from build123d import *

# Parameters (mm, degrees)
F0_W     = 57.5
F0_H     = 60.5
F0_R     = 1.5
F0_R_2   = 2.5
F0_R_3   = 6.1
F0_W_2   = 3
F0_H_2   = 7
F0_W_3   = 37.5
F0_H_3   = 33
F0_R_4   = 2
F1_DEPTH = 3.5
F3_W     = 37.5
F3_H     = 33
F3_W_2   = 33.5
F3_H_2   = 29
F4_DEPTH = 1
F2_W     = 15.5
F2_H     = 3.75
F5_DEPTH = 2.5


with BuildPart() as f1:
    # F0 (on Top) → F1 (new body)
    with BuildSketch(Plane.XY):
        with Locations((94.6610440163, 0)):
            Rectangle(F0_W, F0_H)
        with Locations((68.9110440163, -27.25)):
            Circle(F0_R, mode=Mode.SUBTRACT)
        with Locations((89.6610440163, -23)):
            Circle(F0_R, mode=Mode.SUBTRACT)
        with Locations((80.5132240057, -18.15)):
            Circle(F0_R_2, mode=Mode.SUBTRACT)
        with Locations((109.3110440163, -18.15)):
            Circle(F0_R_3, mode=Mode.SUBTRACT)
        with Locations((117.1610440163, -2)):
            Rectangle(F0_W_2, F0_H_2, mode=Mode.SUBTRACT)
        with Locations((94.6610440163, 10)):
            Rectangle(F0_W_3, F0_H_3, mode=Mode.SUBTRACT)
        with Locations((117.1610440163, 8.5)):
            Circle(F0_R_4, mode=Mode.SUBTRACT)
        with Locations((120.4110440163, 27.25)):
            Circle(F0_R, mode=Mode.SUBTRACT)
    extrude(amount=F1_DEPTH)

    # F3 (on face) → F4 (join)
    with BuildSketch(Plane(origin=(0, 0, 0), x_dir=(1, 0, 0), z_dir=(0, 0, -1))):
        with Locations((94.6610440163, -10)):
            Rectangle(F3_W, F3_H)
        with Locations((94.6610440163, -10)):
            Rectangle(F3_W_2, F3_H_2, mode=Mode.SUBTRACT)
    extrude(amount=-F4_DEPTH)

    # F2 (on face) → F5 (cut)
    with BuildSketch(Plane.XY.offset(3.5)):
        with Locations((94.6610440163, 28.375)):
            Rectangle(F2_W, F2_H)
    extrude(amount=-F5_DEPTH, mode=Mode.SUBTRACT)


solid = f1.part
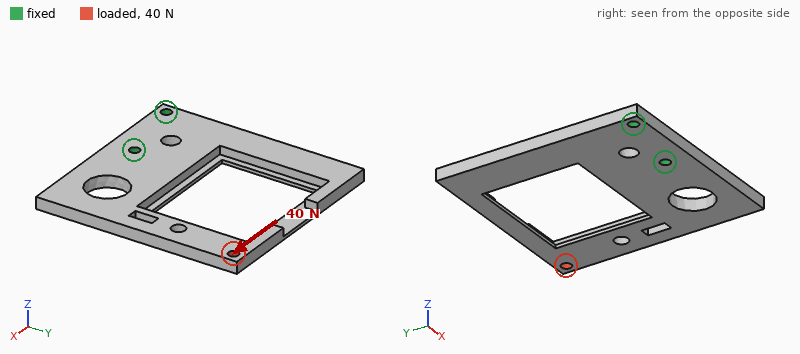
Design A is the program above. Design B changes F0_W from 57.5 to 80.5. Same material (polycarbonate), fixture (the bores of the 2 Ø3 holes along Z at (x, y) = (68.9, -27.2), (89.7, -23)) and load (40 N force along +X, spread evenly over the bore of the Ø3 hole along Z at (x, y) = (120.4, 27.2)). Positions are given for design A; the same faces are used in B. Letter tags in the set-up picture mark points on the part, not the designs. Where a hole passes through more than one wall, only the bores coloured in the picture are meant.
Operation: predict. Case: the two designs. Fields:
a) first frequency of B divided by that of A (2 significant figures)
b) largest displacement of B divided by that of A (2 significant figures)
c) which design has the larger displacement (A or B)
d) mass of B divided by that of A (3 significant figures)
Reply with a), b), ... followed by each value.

a) 0.71
b) 0.61
c) A
d) 1.67
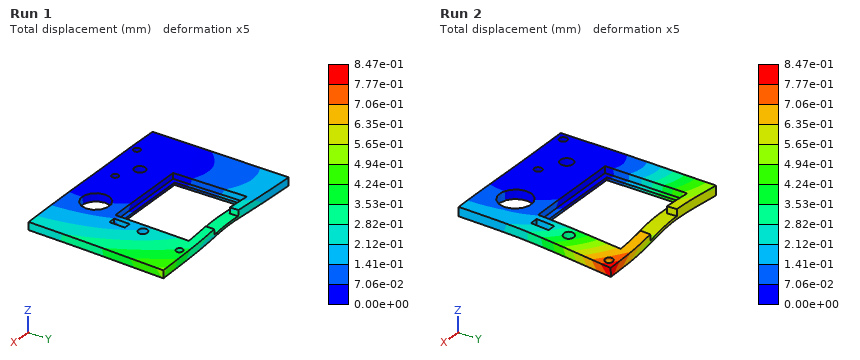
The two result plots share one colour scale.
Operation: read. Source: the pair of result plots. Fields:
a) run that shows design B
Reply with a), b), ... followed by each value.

a) Run 1
